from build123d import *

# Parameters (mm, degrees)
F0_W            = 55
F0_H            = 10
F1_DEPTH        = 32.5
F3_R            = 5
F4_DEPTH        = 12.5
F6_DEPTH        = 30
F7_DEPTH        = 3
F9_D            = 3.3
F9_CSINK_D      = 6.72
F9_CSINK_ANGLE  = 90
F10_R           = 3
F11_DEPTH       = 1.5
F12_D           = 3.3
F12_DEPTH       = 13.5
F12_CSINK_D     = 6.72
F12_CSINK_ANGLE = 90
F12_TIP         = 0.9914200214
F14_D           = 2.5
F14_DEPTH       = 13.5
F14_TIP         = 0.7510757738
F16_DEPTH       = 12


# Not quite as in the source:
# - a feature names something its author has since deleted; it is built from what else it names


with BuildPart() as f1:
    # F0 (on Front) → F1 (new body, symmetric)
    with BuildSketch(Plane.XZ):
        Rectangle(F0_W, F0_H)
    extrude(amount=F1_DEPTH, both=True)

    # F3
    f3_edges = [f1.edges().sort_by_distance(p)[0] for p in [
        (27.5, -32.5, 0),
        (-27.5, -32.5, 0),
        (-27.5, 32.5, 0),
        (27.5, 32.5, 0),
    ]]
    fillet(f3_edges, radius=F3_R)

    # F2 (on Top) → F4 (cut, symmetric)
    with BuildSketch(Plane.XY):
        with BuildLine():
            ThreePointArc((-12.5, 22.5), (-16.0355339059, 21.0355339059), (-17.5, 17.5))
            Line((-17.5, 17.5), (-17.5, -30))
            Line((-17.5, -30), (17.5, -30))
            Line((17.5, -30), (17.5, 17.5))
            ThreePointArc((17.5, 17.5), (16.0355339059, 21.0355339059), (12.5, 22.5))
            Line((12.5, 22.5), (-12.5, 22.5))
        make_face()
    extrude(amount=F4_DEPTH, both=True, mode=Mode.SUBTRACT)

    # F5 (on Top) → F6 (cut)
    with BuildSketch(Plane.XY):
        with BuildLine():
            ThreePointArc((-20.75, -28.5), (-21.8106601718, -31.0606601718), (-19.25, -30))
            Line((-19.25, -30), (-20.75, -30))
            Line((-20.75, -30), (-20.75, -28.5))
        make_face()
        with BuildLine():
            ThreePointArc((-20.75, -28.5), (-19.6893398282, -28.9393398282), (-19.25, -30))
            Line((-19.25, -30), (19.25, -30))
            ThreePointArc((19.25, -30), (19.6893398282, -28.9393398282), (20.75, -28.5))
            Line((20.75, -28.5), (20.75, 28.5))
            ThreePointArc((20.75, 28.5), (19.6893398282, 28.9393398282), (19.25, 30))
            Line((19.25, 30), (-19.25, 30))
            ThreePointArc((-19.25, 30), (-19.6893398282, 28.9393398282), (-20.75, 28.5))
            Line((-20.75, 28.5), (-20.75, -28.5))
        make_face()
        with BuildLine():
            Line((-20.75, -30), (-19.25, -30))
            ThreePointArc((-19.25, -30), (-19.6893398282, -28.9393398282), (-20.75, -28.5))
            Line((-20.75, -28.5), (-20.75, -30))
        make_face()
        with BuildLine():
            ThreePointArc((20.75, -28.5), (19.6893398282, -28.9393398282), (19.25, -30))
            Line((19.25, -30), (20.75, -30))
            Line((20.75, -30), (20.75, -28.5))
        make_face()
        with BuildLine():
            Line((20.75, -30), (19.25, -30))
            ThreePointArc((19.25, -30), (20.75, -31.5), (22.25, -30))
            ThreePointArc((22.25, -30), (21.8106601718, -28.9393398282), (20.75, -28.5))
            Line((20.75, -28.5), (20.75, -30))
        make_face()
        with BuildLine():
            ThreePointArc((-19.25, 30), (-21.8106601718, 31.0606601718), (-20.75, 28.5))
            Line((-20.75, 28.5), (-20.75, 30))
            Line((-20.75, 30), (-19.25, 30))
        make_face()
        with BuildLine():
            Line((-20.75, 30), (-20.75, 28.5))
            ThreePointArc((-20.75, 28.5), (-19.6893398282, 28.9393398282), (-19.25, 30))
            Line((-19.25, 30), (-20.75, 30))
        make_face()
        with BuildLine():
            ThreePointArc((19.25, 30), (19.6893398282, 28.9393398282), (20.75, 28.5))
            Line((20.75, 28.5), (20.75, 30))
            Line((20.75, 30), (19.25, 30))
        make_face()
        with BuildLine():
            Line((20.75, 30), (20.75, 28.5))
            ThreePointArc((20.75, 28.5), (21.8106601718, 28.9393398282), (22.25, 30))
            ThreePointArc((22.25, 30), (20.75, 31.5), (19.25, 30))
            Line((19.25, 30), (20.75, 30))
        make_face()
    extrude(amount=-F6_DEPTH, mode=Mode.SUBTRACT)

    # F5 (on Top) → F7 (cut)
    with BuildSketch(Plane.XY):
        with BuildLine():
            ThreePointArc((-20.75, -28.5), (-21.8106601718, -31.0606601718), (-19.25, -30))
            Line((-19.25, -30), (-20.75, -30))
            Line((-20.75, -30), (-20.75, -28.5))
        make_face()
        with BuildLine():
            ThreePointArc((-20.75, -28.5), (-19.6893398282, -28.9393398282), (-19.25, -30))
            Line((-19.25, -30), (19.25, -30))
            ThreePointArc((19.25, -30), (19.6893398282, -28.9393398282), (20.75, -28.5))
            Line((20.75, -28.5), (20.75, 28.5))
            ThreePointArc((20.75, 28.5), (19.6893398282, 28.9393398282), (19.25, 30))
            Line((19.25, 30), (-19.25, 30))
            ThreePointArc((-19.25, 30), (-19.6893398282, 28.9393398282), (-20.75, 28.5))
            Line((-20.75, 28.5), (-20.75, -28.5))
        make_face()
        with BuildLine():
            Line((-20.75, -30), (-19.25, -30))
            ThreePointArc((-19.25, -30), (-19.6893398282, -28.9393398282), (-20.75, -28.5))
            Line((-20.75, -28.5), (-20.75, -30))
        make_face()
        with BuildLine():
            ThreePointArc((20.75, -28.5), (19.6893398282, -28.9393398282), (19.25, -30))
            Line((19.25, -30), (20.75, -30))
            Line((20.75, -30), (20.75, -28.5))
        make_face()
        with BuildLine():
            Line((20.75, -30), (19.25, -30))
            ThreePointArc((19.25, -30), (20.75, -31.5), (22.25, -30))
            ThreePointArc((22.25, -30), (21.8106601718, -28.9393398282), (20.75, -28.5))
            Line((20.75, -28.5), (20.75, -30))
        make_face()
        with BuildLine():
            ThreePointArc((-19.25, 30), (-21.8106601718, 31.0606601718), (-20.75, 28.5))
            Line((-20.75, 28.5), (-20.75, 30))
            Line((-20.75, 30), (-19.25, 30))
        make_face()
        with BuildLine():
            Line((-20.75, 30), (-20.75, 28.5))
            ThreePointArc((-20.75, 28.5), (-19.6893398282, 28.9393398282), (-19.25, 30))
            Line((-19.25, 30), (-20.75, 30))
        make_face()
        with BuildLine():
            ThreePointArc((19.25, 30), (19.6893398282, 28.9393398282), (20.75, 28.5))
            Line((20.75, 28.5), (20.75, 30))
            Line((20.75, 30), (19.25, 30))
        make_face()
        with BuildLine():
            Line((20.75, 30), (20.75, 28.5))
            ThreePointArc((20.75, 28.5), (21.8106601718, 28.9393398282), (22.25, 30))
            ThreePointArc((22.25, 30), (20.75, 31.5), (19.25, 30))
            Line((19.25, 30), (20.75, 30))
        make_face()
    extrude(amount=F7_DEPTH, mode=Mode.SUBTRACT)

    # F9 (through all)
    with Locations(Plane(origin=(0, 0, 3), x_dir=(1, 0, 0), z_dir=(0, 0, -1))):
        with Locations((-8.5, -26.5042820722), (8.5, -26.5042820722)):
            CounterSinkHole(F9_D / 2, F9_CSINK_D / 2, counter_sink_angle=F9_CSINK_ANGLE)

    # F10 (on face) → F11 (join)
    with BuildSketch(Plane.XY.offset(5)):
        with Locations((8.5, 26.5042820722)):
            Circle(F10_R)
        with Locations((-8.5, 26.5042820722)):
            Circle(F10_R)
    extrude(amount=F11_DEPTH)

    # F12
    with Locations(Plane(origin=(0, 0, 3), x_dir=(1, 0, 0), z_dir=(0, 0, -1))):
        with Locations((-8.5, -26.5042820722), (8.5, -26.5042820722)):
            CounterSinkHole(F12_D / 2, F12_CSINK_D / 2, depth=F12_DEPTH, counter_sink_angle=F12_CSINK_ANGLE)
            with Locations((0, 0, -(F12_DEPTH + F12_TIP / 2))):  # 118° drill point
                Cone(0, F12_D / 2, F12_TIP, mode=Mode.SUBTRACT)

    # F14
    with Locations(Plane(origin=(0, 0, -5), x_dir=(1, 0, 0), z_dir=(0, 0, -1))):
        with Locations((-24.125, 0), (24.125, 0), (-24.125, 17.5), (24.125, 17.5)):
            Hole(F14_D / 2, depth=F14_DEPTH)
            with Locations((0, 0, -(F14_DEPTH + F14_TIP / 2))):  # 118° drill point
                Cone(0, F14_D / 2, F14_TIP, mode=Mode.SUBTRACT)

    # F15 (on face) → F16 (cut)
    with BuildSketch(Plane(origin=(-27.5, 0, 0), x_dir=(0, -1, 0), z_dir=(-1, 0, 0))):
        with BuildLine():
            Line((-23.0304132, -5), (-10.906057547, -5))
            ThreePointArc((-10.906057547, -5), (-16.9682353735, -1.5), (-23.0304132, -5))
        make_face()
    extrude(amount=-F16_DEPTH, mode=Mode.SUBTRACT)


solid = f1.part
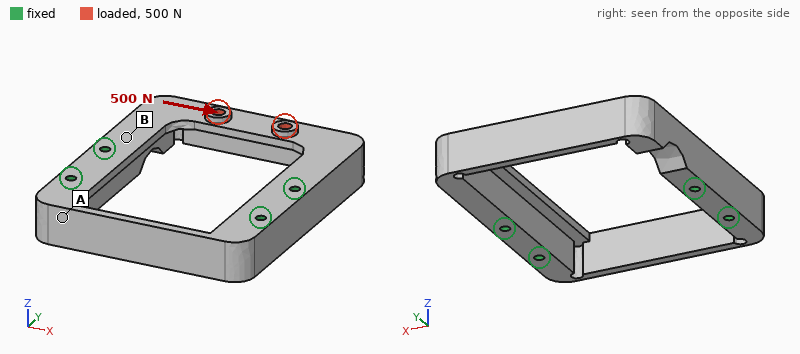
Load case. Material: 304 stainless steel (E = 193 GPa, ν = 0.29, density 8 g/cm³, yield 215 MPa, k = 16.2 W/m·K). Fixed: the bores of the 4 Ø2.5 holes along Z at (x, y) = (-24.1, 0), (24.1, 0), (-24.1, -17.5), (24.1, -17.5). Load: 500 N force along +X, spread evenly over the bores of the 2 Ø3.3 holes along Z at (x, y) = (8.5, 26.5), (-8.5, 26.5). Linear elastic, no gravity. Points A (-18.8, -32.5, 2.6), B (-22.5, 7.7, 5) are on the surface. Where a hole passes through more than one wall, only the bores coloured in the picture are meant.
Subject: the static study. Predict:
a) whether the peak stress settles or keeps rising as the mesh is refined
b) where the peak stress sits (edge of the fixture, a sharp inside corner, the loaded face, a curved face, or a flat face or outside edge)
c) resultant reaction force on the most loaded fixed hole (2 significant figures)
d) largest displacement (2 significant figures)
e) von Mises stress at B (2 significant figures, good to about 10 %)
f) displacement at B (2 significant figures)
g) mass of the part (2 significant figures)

keeps rising
a sharp inside corner
400 N
16 µm
18 MPa
2.9 µm
91 g
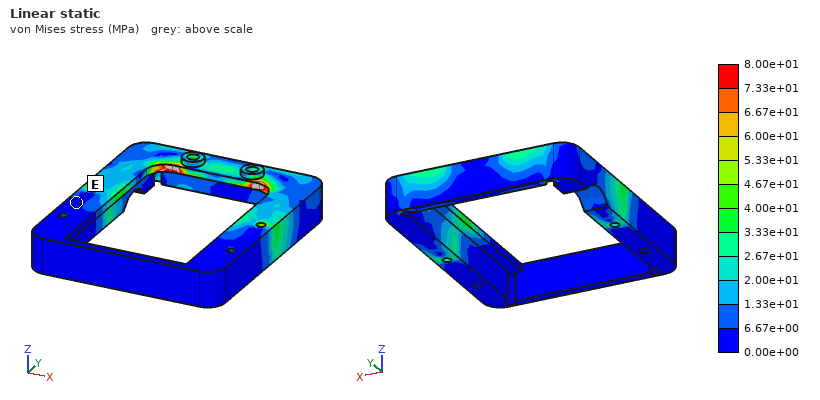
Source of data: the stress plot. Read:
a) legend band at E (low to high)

0.00e+00 to 6.67e+00 MPa
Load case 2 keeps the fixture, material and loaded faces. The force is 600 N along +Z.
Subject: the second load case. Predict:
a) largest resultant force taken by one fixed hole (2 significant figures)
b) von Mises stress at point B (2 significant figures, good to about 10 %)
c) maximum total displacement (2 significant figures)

390 N
45 MPa
58 µm
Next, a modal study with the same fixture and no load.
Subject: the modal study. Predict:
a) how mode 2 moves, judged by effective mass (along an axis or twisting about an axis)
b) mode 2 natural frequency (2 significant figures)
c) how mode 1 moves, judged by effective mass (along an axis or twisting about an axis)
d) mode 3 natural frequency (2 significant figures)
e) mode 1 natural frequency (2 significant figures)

along X
5400 Hz
along Z
5900 Hz
4500 Hz
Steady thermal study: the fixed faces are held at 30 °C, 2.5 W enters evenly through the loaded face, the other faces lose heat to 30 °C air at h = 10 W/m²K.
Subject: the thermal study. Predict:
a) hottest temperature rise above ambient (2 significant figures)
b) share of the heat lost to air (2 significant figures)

54 K
36 %
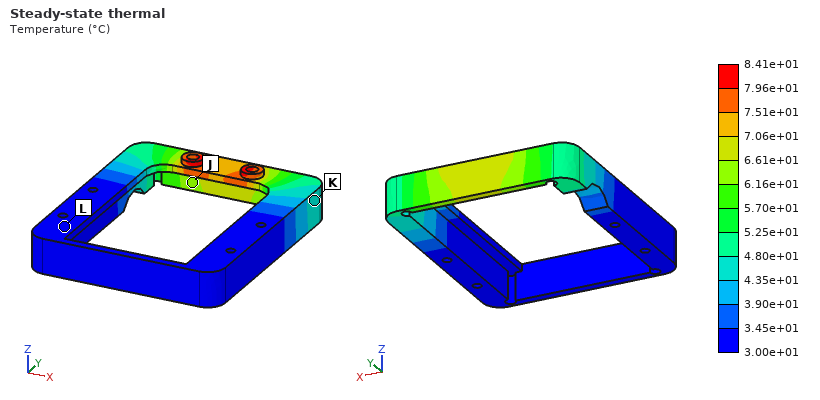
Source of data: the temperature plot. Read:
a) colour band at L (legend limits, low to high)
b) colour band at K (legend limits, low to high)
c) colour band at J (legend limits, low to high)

3.00e+01 to 3.45e+01 °C
4.35e+01 to 4.80e+01 °C
6.16e+01 to 6.61e+01 °C
